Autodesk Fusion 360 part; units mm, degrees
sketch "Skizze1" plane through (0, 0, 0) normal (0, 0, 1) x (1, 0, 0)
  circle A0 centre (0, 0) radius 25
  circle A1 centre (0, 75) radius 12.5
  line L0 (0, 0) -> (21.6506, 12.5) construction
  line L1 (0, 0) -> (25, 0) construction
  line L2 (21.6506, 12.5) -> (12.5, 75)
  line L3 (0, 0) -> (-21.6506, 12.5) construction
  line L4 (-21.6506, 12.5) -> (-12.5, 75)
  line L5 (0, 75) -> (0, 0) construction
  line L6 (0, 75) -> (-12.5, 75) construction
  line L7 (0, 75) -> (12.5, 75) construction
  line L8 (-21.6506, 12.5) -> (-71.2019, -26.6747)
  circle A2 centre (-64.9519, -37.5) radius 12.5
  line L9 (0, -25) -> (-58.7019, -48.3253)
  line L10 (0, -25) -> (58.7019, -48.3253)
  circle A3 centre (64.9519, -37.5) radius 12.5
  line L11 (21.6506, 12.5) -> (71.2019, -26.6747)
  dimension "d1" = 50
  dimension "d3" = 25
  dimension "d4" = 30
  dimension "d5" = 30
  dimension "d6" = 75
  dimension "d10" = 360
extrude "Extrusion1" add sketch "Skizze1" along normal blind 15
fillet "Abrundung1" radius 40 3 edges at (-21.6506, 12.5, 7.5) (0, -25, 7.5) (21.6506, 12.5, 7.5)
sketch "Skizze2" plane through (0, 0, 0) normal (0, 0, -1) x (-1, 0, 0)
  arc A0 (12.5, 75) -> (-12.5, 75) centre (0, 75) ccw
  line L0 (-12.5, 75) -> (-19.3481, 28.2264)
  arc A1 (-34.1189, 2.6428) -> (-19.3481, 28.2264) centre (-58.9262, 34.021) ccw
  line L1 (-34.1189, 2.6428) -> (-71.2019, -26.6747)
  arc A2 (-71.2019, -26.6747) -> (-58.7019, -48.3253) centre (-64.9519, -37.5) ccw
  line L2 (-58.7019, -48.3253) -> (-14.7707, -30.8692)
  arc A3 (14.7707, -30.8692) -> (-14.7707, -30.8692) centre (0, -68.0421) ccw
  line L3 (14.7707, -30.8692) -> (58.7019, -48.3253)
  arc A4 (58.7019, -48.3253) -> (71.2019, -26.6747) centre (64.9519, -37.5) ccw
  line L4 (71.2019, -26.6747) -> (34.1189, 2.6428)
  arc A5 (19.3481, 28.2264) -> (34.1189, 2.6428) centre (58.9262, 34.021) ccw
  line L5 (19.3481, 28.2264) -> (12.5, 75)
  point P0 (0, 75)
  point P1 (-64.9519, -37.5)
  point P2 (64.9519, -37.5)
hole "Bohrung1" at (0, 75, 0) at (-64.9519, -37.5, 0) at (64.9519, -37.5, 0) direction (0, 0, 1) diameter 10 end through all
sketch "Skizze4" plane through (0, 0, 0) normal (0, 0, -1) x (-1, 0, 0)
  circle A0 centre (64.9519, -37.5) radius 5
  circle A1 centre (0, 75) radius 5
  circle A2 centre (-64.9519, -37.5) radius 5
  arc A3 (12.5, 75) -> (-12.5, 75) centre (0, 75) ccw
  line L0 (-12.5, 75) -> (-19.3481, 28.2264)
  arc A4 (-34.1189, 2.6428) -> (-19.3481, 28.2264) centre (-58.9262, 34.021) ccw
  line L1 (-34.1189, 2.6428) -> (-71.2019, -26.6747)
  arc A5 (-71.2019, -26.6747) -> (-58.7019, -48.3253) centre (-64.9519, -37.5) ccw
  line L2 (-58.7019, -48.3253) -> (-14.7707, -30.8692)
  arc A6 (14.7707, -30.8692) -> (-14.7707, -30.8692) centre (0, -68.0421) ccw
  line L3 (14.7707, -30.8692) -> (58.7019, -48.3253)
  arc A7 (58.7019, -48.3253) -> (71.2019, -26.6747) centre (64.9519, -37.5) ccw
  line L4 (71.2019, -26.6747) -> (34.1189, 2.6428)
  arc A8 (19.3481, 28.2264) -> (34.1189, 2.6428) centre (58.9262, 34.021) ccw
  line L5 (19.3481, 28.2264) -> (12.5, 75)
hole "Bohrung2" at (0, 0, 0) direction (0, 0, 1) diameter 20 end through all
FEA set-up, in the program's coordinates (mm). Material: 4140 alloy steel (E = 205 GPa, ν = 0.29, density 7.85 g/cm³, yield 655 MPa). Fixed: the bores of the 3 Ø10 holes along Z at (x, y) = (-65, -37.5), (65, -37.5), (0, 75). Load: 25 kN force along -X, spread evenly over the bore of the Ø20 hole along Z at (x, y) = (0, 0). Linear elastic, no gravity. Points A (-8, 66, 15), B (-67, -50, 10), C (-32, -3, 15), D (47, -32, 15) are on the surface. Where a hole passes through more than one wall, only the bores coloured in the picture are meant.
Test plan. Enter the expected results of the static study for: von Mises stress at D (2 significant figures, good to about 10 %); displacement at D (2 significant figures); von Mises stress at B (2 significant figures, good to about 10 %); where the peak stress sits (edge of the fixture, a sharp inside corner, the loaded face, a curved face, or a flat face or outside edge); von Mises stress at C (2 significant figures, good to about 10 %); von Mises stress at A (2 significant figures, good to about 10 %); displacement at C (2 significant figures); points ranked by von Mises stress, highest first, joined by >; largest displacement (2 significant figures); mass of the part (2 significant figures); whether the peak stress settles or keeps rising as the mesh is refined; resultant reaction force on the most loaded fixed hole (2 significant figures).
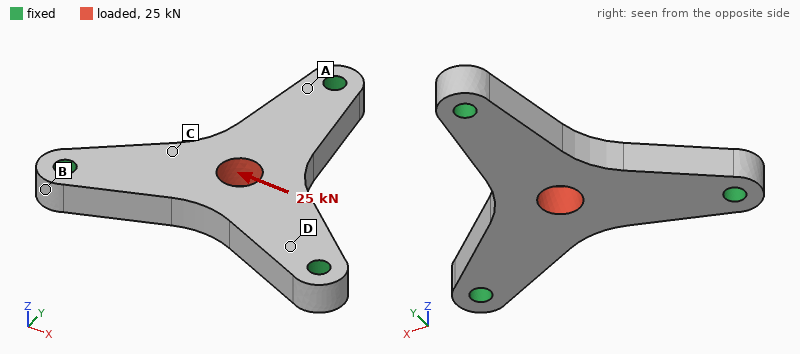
31 MPa
2.9 µm
6.9 MPa
edge of the fixture
23 MPa
12 MPa
9.8 µm
D > C > A > B
16 µm
880 g
keeps rising
13 kN
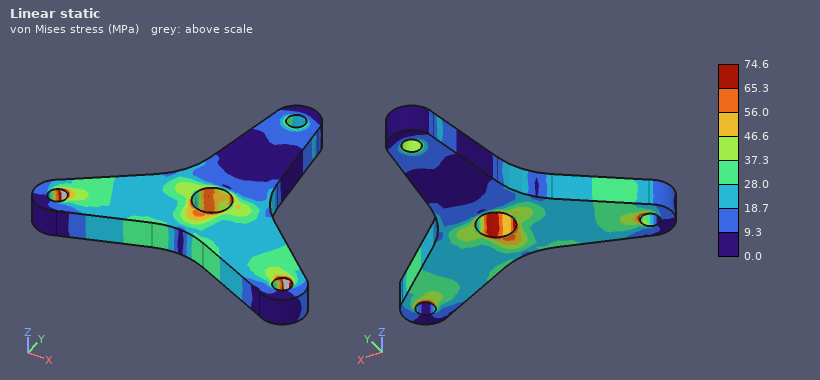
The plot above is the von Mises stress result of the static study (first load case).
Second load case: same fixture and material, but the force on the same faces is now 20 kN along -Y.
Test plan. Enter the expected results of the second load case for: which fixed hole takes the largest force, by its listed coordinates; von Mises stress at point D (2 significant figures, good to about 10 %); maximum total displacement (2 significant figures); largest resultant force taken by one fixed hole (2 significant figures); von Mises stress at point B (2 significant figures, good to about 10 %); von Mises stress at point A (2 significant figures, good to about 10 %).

(0, 75)
17 MPa
13 µm
12 kN
7.7 MPa
27 MPa
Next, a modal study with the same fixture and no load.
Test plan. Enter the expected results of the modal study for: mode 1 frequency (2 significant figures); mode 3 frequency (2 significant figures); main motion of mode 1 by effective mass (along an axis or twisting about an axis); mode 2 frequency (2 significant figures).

3700 Hz
7700 Hz
along Z
7700 Hz
